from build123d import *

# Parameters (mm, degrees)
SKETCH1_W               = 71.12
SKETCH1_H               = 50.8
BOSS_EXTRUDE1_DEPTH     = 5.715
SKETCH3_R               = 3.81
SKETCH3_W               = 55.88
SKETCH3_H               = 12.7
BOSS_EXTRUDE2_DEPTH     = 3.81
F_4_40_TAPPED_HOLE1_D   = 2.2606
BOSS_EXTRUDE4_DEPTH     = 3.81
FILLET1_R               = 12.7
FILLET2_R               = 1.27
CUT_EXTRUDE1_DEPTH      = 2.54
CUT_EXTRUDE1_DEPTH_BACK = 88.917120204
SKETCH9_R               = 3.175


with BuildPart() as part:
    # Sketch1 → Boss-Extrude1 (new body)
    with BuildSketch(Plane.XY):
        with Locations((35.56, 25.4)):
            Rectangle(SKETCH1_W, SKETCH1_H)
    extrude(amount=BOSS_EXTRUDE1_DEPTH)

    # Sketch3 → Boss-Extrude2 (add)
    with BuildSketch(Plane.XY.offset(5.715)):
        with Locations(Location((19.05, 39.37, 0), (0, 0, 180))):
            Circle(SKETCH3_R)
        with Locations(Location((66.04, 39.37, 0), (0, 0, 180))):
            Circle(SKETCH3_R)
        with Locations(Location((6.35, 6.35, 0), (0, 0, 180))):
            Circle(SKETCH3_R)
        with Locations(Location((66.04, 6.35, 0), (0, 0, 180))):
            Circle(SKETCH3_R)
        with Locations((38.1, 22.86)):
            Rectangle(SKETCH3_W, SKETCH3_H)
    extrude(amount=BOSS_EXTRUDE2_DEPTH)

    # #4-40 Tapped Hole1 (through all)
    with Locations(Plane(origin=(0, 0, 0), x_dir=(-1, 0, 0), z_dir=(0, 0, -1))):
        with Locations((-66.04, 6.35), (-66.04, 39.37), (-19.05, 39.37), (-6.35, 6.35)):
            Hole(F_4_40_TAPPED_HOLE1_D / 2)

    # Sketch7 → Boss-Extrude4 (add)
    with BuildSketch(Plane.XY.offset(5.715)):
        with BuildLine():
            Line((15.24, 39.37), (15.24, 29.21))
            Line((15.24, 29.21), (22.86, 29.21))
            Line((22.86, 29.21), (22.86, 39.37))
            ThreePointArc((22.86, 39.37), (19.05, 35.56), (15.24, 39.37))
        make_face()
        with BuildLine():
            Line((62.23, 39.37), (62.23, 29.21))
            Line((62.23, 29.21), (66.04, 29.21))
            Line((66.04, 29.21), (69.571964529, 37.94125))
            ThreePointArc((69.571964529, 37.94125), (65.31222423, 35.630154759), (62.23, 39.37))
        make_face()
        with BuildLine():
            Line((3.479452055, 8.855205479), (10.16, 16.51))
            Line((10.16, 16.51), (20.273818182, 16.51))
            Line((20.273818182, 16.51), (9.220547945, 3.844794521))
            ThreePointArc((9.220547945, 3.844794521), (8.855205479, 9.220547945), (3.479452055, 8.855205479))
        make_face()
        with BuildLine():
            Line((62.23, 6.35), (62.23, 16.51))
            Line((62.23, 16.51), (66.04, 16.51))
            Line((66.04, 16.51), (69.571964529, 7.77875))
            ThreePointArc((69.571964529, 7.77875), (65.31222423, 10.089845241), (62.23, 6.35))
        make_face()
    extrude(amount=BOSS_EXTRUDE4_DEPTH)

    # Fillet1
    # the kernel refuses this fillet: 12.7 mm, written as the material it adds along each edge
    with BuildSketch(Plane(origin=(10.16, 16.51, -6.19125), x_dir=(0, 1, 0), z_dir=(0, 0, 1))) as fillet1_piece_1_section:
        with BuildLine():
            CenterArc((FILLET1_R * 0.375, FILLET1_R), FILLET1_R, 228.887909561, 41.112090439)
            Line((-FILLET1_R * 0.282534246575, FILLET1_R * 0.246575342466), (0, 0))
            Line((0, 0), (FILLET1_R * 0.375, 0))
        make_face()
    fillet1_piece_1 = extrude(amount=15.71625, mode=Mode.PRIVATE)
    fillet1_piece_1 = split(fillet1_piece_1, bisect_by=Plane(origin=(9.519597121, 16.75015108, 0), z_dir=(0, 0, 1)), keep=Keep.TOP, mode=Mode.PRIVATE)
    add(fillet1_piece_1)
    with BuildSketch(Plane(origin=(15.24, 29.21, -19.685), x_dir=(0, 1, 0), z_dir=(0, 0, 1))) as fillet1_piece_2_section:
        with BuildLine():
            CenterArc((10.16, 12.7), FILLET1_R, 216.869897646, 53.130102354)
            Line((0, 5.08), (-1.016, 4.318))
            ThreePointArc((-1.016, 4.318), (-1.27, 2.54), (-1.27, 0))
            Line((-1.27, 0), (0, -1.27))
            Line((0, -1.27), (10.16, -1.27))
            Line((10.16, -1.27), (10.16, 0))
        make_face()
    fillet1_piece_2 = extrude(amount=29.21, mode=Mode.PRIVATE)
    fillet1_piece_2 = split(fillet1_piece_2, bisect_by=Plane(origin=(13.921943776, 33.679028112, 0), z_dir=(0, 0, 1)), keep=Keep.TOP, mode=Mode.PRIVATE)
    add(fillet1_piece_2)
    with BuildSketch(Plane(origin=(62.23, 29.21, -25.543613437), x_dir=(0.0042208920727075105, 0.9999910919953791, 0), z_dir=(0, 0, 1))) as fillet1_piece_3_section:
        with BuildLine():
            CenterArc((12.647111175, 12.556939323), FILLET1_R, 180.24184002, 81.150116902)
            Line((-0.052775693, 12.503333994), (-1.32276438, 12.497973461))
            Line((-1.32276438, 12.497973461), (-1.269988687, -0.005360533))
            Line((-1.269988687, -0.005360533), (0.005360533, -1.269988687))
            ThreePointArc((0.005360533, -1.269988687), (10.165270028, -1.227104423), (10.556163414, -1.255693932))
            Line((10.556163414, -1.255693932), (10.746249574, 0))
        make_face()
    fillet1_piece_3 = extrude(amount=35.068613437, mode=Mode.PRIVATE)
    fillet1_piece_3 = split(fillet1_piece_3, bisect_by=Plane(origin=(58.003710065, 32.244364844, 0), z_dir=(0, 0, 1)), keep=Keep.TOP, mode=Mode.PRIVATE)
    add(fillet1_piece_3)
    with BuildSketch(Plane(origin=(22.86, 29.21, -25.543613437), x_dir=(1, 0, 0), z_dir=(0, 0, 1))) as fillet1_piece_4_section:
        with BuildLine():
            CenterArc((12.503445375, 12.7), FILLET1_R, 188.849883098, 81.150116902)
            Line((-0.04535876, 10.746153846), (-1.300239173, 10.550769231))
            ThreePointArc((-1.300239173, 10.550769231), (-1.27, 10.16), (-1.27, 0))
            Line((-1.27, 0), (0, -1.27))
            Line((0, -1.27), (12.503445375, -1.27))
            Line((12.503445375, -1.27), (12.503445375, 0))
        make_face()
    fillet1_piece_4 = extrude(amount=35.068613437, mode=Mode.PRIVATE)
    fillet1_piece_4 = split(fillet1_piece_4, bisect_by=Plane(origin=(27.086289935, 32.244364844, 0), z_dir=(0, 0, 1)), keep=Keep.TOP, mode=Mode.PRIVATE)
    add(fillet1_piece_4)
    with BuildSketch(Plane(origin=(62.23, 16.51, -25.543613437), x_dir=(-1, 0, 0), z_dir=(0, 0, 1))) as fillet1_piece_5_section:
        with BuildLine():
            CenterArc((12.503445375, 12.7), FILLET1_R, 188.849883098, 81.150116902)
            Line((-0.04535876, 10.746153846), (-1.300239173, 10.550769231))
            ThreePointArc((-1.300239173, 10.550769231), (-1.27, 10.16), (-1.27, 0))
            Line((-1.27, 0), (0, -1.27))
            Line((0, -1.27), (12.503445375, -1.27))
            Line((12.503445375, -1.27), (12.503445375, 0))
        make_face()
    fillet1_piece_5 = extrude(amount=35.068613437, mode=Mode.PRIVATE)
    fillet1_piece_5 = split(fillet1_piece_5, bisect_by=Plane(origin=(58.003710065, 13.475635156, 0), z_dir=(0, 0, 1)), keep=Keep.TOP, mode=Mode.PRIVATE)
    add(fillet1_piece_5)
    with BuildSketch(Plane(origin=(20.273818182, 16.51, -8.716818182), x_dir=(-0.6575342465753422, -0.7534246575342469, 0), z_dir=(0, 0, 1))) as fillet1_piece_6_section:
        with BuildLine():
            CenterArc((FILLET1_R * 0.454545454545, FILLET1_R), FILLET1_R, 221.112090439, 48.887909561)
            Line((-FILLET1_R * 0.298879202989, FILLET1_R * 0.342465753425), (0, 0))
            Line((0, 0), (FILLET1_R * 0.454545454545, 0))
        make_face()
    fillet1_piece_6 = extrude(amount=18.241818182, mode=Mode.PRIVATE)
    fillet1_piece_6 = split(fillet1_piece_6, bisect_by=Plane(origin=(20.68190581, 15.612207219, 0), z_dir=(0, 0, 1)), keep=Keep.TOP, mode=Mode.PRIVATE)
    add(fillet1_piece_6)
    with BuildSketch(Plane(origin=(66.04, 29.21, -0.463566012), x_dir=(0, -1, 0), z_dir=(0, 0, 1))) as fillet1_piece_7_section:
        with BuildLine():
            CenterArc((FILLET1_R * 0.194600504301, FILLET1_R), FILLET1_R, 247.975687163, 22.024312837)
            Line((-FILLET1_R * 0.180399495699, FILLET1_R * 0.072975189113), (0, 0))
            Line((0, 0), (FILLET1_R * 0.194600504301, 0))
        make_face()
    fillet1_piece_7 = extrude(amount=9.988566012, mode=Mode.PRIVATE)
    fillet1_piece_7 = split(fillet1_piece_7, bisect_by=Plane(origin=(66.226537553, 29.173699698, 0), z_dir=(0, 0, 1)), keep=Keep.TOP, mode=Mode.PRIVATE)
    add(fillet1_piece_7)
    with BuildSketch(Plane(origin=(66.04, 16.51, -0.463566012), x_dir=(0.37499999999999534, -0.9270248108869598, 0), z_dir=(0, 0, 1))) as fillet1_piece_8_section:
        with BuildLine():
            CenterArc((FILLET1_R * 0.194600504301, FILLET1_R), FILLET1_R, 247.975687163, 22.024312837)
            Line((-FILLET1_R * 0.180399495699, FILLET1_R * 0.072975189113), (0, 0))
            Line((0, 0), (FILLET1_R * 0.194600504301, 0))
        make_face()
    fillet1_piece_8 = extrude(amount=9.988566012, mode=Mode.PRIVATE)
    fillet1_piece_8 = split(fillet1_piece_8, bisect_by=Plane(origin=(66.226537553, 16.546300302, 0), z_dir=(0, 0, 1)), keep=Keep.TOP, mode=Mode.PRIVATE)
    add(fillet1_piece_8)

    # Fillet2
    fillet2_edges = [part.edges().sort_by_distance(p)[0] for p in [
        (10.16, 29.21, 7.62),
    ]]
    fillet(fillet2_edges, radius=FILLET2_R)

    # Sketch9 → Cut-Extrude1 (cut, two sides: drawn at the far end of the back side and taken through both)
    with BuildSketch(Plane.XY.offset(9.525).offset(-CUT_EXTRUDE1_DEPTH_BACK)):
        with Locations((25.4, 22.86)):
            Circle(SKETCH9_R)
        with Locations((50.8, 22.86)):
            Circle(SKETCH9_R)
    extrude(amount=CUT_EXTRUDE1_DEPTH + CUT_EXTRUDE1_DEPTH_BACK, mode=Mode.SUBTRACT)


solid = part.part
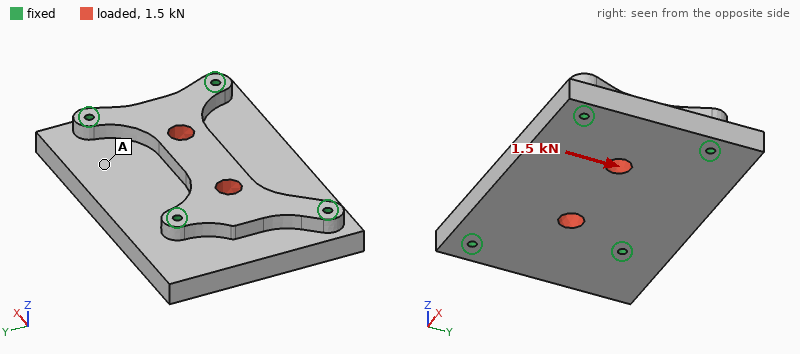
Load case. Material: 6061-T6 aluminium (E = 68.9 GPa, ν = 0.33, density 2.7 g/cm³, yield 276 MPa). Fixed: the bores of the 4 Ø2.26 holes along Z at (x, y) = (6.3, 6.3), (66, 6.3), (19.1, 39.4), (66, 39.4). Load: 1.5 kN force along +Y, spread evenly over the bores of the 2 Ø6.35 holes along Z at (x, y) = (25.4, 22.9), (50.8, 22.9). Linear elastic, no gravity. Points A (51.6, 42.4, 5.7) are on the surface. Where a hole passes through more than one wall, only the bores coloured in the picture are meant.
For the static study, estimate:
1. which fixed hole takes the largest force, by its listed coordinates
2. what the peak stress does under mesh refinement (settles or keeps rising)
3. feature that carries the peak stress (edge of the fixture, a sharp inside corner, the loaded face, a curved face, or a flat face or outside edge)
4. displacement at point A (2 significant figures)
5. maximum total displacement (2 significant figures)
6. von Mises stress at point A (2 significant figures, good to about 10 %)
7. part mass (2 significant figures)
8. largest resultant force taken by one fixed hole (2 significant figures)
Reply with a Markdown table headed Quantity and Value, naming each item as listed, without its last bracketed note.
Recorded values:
| Quantity | Value |
|---|---|
| which fixed hole takes the largest force, by its listed coordinates | (19.1, 39.4) |
| what the peak stress does under mesh refinement | keeps rising |
| feature that carries the peak stress | edge of the fixture |
| displacement at point A | 1.3 µm |
| maximum total displacement | 2.5 µm |
| von Mises stress at point A | 1.8 MPa |
| part mass | 66 g |
| largest resultant force taken by one fixed hole | 630 N |
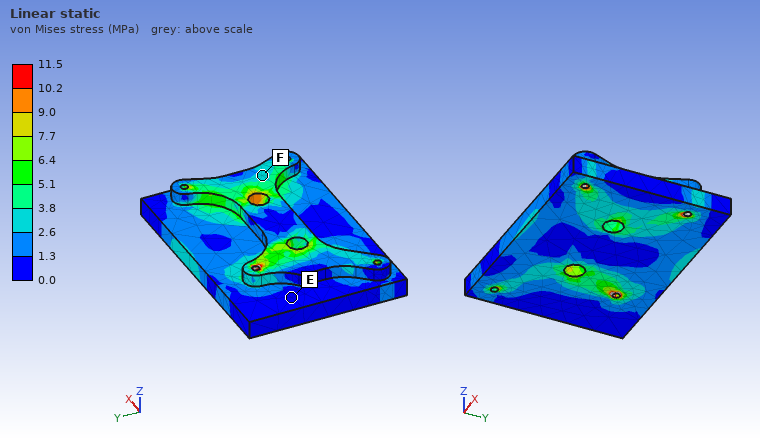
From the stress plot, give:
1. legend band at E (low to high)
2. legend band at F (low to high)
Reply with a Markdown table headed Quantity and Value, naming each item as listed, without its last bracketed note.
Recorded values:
| Quantity | Value |
|---|---|
| legend band at E | 0.0 to 1.3 MPa |
| legend band at F | 2.6 to 3.8 MPa |
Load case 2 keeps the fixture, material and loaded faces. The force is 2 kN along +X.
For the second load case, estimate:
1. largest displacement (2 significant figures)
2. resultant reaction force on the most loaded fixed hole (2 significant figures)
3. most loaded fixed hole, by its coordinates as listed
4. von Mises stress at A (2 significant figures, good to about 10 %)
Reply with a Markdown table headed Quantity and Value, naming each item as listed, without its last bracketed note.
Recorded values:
| Quantity | Value |
|---|---|
| largest displacement | 2.5 µm |
| resultant reaction force on the most loaded fixed hole | 610 N |
| most loaded fixed hole, by its coordinates as listed | (19.1, 39.4) |
| von Mises stress at A | 2.0 MPa |
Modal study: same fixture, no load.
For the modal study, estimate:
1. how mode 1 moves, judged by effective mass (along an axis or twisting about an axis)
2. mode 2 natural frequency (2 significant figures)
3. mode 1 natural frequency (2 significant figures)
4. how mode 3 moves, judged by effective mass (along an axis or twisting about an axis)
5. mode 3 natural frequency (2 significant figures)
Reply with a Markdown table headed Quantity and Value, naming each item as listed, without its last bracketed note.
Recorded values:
| Quantity | Value |
|---|---|
| how mode 1 moves, judged by effective mass | along Z |
| mode 2 natural frequency | 13 kHz |
| mode 1 natural frequency | 9500 Hz |
| how mode 3 moves, judged by effective mass | along Z |
| mode 3 natural frequency | 14 kHz |
